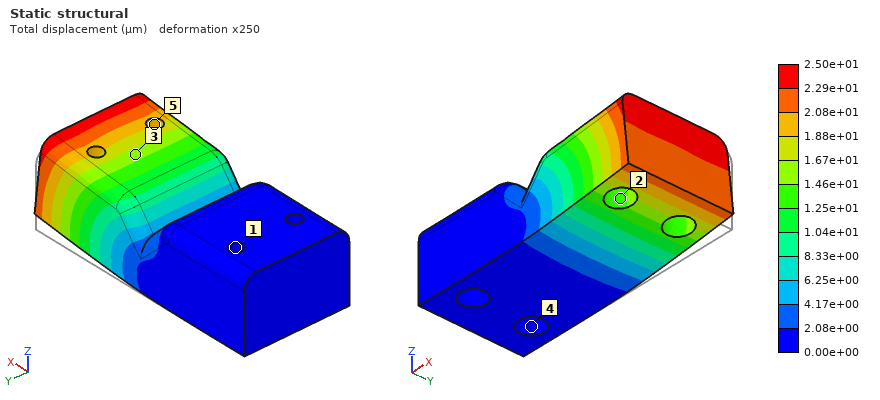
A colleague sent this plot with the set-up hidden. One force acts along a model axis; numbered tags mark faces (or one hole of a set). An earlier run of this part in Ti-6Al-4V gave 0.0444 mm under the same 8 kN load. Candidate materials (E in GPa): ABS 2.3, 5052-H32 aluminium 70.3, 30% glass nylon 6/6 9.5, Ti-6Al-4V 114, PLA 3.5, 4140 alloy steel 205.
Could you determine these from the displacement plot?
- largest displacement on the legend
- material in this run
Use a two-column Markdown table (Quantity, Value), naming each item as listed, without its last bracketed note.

| Quantity | Value |
|---|---|
| largest displacement on the legend | 2.50e+01 µm |
| material in this run | 4140 alloy steel |
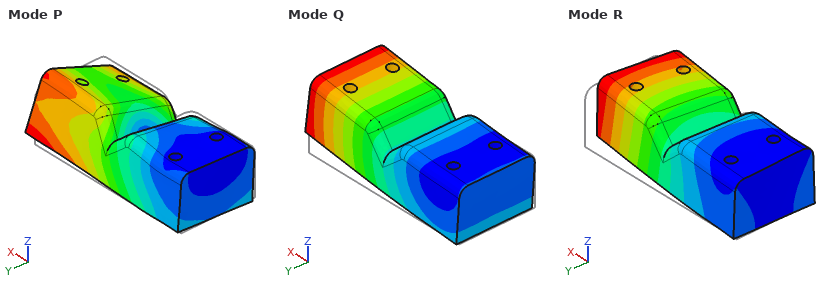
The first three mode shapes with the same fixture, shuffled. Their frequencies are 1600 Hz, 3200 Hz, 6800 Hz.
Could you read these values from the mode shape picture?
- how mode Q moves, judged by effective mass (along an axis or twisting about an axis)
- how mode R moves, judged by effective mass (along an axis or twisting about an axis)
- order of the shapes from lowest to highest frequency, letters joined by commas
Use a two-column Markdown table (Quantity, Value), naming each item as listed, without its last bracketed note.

| Quantity | Value |
|---|---|
| how mode Q moves, judged by effective mass | along Z |
| how mode R moves, judged by effective mass | along Y |
| order of the shapes from lowest to highest frequency, letters joined by commas | Q, R, P |
